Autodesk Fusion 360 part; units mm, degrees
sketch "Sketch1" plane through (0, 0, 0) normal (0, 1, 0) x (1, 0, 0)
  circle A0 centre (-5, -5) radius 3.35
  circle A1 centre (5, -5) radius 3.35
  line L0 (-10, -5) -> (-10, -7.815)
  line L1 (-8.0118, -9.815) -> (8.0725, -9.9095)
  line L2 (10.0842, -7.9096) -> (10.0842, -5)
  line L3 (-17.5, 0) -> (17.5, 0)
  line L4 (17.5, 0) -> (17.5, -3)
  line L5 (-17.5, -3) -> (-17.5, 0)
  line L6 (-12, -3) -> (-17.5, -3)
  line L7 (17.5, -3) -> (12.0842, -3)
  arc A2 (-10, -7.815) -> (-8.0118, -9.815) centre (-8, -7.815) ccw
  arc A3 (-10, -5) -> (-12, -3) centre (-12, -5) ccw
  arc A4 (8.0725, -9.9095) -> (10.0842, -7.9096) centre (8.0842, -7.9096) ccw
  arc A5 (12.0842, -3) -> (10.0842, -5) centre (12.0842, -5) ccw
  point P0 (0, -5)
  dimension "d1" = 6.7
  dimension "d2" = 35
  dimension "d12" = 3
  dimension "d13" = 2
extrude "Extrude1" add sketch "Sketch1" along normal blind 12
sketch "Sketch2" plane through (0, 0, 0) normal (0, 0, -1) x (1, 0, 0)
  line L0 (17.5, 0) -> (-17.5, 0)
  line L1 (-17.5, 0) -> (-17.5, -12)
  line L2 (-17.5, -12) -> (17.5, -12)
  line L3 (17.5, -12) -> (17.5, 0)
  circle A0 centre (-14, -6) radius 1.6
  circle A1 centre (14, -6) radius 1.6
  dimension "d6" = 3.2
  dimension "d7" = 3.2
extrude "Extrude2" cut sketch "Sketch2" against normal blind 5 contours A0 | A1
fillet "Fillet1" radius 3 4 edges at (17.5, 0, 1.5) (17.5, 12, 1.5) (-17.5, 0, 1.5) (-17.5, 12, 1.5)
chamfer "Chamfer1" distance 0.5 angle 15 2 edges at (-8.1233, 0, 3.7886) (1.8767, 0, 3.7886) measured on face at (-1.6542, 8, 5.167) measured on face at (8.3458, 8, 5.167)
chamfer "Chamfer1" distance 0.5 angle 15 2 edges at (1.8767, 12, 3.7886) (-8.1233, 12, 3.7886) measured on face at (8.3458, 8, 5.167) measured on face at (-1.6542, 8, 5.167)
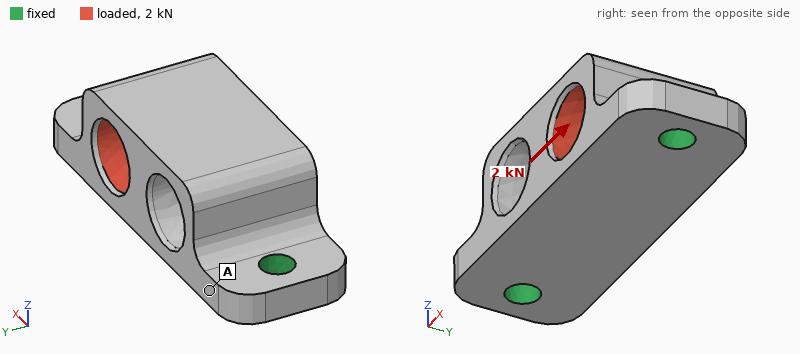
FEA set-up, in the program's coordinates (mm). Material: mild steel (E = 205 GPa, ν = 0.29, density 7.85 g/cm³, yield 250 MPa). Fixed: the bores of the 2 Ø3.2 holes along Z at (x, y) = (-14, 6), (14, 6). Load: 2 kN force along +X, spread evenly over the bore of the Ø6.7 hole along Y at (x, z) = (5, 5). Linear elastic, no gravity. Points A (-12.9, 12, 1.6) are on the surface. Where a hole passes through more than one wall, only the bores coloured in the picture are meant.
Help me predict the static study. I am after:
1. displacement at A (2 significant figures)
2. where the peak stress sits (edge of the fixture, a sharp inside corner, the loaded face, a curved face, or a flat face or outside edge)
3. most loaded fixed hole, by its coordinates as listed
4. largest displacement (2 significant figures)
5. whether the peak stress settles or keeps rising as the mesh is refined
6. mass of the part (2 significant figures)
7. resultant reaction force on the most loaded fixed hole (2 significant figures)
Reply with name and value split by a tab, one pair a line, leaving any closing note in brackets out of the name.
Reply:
displacement at A	0.73 µm
where the peak stress sits	edge of the fixture
most loaded fixed hole, by its coordinates as listed	(14, 6)
largest displacement	4.8 µm
whether the peak stress settles or keeps rising as the mesh is refined	keeps rising
mass of the part	16 g
resultant reaction force on the most loaded fixed hole	1.3 kN
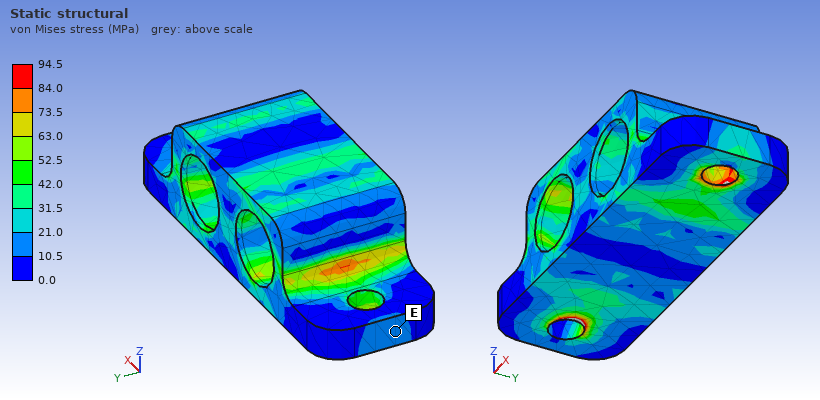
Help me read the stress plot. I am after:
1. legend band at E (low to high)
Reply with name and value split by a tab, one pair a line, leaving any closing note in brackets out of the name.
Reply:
legend band at E	10.5 to 21.0 MPa
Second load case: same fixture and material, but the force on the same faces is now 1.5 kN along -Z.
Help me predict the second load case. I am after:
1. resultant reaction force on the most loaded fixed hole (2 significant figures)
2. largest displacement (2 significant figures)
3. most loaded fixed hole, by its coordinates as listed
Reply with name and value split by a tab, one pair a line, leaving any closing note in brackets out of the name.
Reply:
resultant reaction force on the most loaded fixed hole	1.1 kN
largest displacement	8.6 µm
most loaded fixed hole, by its coordinates as listed	(14, 6)
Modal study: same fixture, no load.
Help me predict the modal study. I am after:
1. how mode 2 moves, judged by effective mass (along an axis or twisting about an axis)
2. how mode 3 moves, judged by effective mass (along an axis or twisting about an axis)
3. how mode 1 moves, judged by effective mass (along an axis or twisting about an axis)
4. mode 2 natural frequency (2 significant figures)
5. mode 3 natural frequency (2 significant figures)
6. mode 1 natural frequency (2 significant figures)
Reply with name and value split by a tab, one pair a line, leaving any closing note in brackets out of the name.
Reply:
how mode 2 moves, judged by effective mass	along Z
how mode 3 moves, judged by effective mass	along Y
how mode 1 moves, judged by effective mass	along Y
mode 2 natural frequency	22 kHz
mode 3 natural frequency	32 kHz
mode 1 natural frequency	16 kHz
